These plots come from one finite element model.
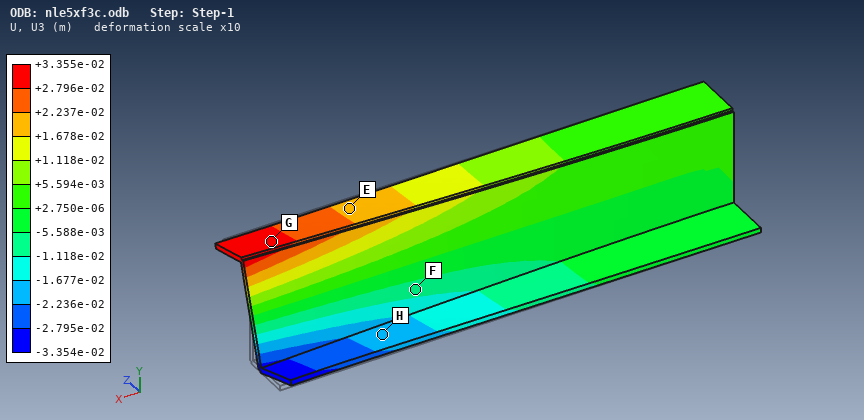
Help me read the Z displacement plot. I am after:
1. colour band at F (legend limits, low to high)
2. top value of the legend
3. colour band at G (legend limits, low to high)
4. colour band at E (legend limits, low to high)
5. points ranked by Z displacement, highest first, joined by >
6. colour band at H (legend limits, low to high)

-1.118e-02 to -5.588e-03 m
+3.355e-02 m
+2.796e-02 to +3.355e-02 m
+1.678e-02 to +2.237e-02 m
G > E > F > H
-2.236e-02 to -1.677e-02 m
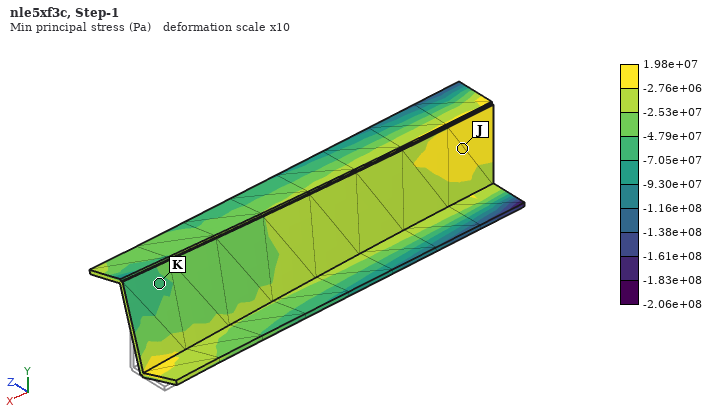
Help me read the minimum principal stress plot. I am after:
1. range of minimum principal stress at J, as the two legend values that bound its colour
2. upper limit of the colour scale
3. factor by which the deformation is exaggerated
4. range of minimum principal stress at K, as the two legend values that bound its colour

-2.76e+06 to 1.98e+07 Pa
1.98e+07 Pa
10
-7.05e+07 to -4.79e+07 Pa
